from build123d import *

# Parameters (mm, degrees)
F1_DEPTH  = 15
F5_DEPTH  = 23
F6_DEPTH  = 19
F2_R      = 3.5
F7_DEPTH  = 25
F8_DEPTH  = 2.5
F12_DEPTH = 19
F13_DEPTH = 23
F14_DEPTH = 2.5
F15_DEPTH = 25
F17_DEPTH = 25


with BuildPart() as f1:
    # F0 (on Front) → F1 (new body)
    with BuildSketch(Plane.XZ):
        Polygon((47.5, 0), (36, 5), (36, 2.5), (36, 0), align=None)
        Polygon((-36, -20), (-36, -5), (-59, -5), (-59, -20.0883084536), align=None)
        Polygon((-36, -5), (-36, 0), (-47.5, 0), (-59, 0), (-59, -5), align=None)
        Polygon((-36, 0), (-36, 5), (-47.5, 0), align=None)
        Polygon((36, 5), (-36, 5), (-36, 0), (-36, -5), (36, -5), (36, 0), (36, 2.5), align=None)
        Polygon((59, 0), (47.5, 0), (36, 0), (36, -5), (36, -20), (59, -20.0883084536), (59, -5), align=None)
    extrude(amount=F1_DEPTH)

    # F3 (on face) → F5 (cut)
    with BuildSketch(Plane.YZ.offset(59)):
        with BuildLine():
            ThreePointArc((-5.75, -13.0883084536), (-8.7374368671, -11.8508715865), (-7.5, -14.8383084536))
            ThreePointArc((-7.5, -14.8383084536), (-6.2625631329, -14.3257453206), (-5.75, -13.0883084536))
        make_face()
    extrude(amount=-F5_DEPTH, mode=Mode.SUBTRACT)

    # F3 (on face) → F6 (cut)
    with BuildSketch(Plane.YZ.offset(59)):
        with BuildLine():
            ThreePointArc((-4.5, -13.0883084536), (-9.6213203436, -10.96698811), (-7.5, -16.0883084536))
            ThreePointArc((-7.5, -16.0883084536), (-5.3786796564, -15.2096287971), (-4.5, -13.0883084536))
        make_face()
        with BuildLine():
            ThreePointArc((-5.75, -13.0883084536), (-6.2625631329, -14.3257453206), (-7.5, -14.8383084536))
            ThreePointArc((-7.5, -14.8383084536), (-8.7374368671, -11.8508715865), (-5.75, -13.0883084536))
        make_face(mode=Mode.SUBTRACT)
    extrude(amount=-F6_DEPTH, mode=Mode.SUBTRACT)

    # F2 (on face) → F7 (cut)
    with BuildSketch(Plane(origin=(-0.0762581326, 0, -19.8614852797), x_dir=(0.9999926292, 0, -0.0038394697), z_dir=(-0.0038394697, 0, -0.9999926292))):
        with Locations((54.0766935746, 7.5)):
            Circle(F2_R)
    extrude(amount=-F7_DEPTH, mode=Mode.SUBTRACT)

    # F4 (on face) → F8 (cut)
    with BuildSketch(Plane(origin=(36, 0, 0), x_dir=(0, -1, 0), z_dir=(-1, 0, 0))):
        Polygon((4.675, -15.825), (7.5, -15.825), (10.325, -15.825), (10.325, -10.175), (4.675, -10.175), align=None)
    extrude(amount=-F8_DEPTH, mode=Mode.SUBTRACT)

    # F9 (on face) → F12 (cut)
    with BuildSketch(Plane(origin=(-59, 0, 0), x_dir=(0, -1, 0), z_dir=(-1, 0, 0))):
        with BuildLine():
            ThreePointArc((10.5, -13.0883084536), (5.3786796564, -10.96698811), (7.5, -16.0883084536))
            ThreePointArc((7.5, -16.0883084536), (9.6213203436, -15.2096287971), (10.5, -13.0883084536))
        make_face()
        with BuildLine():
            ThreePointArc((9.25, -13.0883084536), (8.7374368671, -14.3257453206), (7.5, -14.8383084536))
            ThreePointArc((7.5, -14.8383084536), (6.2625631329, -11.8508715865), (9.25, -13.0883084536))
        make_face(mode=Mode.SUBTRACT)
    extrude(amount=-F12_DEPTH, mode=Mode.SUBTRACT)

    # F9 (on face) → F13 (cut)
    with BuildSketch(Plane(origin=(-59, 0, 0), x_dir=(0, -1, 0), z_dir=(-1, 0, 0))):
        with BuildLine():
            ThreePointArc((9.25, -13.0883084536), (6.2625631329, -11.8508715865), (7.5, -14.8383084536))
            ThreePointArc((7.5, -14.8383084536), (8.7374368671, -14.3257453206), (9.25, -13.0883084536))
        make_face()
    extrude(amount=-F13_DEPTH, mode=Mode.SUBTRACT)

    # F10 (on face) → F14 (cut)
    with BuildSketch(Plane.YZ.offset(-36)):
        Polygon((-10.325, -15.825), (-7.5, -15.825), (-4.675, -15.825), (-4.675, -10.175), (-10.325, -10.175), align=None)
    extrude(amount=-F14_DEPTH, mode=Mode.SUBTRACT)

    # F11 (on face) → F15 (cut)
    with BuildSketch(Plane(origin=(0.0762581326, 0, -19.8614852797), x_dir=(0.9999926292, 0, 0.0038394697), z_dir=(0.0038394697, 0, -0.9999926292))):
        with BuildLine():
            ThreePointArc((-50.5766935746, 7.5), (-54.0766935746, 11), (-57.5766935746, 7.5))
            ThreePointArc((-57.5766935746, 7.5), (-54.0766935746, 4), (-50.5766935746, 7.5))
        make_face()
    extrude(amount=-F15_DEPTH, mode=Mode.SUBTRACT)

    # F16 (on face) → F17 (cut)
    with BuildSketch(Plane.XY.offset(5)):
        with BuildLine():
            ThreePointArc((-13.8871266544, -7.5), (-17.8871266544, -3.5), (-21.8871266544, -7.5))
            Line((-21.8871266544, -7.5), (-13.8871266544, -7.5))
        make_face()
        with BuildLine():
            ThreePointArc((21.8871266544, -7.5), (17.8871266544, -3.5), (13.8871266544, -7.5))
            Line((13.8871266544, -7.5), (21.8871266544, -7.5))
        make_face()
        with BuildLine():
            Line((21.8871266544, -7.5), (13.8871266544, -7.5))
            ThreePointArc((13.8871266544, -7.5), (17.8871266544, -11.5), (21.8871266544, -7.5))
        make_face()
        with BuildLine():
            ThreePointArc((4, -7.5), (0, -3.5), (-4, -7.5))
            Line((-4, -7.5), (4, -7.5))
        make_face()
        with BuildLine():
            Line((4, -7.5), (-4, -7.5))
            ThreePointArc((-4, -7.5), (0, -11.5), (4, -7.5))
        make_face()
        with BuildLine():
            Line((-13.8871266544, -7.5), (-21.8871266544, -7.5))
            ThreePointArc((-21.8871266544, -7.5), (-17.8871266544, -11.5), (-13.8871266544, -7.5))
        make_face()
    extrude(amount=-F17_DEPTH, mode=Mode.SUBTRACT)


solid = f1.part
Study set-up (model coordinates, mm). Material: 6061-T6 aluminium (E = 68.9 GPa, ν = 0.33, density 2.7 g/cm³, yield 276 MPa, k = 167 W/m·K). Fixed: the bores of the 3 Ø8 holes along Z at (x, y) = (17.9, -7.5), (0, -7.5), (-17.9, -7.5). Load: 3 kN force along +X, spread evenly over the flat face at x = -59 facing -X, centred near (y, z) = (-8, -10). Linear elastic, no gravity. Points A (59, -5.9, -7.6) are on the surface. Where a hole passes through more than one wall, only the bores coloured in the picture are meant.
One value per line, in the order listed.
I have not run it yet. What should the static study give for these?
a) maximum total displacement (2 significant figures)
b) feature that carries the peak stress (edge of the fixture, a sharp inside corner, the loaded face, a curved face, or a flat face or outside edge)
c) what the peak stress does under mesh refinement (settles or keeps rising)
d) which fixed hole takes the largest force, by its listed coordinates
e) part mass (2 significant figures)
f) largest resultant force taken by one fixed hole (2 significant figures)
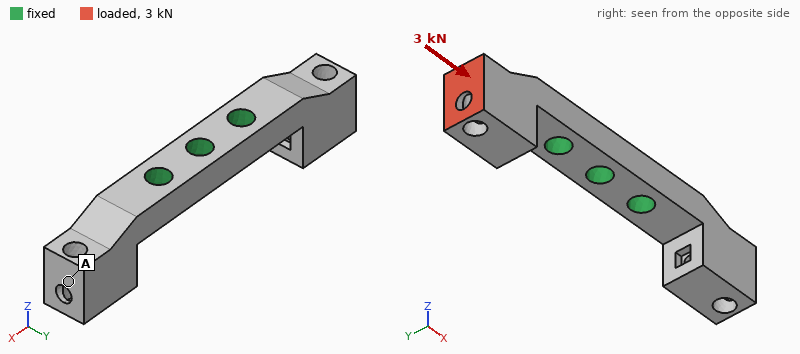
0.27 mm
edge of the fixture
keeps rising
(-17.9, -7.5)
58 g
2.9 kN
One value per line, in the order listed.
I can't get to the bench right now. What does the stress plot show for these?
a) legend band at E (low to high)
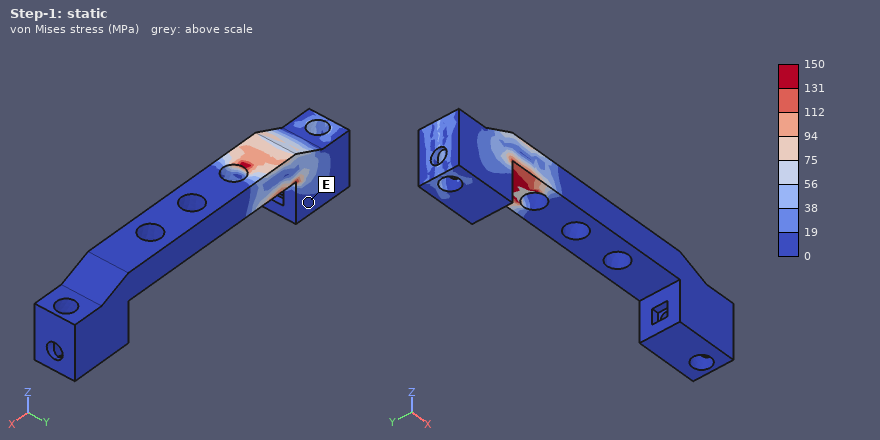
0 to 19 MPa
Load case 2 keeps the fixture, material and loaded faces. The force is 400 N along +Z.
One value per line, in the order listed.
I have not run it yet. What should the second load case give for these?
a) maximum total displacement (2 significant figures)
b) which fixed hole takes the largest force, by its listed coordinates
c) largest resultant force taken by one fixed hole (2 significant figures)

0.11 mm
(-17.9, -7.5)
440 N
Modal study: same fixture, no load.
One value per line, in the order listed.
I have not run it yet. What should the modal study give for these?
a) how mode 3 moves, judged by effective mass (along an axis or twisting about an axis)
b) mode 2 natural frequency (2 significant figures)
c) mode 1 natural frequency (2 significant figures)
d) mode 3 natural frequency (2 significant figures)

along Y
3700 Hz
3700 Hz
4500 Hz
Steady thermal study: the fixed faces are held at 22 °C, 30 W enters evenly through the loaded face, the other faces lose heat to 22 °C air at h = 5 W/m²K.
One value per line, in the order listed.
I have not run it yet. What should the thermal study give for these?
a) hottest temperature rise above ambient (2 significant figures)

44 K
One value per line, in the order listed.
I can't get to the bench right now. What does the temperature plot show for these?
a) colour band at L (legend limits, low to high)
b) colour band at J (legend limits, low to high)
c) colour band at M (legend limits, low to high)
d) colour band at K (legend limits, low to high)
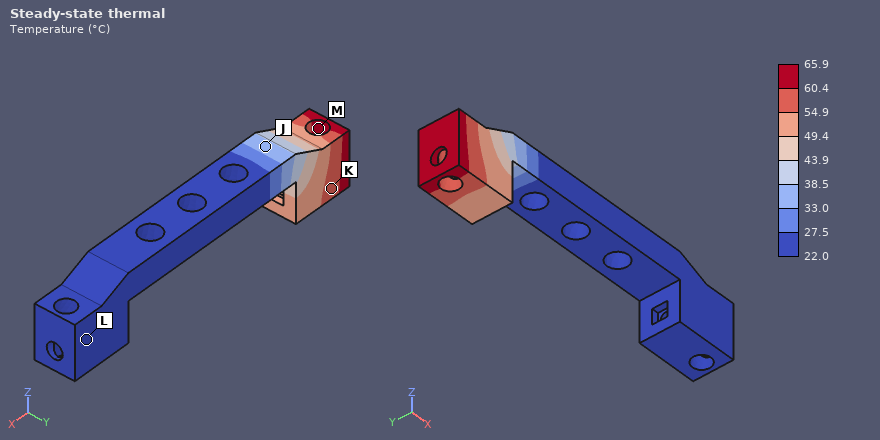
22.0 to 27.5 °C
33.0 to 38.5 °C
60.4 to 65.9 °C
54.9 to 60.4 °C
